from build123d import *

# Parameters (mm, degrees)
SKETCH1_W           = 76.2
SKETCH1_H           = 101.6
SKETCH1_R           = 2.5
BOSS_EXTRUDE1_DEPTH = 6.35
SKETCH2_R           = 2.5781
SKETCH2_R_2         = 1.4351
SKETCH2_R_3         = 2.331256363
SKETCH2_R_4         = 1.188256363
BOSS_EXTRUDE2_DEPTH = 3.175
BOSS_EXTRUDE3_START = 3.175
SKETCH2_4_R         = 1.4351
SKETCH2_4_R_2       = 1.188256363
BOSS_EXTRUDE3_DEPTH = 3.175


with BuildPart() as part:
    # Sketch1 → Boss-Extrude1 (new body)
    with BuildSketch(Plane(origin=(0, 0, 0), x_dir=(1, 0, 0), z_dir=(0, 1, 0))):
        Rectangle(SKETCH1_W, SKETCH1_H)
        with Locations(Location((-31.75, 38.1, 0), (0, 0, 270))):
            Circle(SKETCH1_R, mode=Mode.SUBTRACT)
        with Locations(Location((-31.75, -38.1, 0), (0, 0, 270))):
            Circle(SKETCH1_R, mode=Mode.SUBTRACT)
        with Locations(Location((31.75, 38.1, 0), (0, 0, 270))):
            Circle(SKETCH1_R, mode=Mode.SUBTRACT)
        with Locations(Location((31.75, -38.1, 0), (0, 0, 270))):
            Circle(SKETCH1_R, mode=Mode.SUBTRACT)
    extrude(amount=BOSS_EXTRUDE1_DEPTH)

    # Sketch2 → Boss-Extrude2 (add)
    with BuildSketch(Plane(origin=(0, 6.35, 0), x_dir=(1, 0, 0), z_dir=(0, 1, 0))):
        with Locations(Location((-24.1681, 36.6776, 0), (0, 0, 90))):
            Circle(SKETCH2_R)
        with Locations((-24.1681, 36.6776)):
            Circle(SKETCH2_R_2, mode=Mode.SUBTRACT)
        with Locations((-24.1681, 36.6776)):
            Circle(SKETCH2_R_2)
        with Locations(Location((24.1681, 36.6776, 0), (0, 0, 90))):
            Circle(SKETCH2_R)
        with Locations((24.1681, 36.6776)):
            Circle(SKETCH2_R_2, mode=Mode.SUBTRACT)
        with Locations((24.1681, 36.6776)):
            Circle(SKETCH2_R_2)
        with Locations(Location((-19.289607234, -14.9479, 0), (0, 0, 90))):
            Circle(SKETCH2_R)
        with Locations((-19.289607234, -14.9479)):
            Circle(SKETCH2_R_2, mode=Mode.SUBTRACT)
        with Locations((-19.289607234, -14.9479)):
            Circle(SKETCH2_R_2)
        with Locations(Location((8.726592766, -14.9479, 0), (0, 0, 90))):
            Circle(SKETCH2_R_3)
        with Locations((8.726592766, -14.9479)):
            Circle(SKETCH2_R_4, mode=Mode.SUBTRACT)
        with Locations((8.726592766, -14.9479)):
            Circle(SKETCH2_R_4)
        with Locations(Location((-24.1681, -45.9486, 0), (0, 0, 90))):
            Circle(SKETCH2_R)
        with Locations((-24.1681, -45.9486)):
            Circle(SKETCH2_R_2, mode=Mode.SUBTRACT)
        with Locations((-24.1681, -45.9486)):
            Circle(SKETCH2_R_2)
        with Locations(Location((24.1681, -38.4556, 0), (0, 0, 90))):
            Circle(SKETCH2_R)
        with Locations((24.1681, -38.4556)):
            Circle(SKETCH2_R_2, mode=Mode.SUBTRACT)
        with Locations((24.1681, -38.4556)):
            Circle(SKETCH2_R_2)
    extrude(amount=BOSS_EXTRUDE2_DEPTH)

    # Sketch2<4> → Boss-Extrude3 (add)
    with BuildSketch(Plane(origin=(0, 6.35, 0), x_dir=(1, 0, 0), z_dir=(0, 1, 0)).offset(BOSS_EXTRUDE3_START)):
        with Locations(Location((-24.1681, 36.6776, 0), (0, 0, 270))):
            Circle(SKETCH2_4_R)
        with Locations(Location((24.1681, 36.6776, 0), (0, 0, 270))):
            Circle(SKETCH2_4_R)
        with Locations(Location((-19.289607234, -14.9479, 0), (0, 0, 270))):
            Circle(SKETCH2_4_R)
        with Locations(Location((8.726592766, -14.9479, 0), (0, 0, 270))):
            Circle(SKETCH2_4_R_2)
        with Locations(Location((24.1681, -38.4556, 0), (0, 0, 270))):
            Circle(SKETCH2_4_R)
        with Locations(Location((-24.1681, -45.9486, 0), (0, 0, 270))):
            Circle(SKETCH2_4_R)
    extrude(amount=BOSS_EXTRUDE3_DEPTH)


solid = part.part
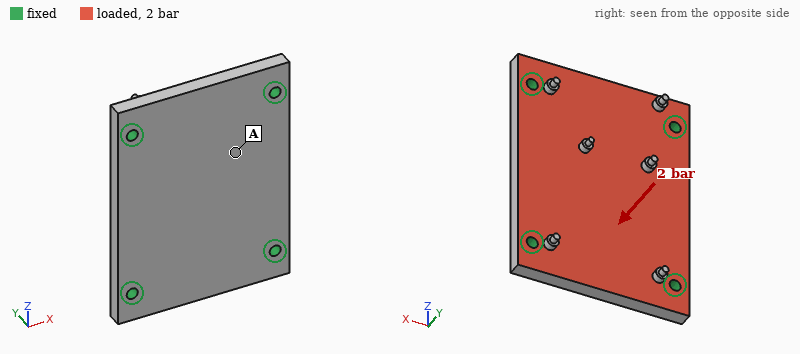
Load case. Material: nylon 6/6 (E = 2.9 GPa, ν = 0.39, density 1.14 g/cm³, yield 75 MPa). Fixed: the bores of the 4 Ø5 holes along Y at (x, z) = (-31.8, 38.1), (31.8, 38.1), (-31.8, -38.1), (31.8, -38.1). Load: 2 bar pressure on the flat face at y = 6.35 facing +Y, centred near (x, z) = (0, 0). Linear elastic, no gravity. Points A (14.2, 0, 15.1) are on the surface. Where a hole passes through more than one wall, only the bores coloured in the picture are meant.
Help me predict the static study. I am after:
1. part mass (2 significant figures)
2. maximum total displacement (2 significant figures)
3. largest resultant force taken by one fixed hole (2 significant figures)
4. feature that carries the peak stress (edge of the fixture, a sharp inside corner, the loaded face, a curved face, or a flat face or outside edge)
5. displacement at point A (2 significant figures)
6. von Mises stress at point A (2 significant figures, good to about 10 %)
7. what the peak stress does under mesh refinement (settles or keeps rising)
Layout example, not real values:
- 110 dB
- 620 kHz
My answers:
- 56 g
- 0.53 mm
- 380 N
- edge of the fixture
- 0.41 mm
- 5.7 MPa
- keeps rising
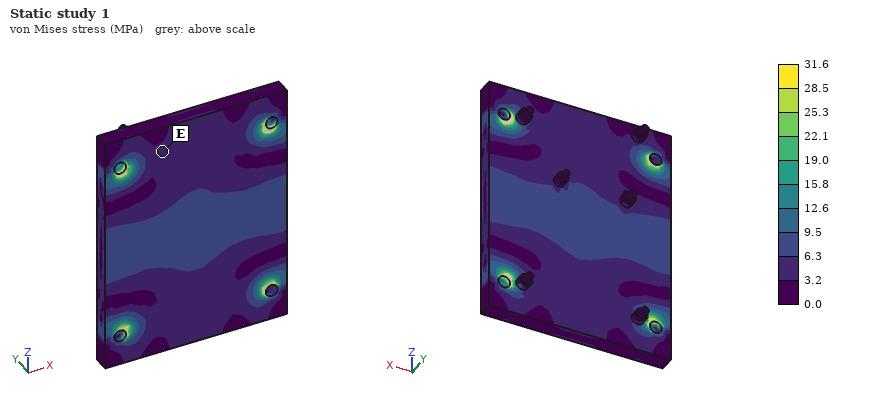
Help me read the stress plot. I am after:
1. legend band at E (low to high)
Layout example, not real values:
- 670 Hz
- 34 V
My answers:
- 3.2 to 6.3 MPa
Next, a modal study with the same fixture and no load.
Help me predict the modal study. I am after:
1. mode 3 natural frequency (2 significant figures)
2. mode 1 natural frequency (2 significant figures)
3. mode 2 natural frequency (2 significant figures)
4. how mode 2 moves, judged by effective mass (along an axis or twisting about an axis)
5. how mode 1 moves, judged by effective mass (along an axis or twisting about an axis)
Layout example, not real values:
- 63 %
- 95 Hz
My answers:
- 2400 Hz
- 1400 Hz
- 2100 Hz
- twisting about Z
- along Y
